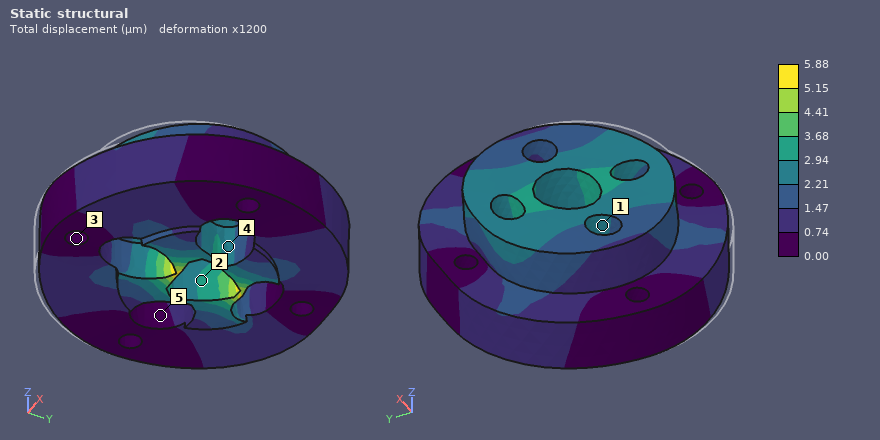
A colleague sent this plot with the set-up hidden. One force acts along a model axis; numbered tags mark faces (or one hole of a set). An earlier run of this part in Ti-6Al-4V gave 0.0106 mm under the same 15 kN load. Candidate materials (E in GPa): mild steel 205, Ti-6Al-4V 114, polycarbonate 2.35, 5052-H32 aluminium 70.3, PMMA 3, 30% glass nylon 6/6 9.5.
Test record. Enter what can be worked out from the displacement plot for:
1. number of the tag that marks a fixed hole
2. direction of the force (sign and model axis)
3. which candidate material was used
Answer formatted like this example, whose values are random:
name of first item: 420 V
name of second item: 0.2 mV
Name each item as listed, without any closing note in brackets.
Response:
number of the tag that marks a fixed hole: 3
direction of the force: +Y
which candidate material was used: mild steel
